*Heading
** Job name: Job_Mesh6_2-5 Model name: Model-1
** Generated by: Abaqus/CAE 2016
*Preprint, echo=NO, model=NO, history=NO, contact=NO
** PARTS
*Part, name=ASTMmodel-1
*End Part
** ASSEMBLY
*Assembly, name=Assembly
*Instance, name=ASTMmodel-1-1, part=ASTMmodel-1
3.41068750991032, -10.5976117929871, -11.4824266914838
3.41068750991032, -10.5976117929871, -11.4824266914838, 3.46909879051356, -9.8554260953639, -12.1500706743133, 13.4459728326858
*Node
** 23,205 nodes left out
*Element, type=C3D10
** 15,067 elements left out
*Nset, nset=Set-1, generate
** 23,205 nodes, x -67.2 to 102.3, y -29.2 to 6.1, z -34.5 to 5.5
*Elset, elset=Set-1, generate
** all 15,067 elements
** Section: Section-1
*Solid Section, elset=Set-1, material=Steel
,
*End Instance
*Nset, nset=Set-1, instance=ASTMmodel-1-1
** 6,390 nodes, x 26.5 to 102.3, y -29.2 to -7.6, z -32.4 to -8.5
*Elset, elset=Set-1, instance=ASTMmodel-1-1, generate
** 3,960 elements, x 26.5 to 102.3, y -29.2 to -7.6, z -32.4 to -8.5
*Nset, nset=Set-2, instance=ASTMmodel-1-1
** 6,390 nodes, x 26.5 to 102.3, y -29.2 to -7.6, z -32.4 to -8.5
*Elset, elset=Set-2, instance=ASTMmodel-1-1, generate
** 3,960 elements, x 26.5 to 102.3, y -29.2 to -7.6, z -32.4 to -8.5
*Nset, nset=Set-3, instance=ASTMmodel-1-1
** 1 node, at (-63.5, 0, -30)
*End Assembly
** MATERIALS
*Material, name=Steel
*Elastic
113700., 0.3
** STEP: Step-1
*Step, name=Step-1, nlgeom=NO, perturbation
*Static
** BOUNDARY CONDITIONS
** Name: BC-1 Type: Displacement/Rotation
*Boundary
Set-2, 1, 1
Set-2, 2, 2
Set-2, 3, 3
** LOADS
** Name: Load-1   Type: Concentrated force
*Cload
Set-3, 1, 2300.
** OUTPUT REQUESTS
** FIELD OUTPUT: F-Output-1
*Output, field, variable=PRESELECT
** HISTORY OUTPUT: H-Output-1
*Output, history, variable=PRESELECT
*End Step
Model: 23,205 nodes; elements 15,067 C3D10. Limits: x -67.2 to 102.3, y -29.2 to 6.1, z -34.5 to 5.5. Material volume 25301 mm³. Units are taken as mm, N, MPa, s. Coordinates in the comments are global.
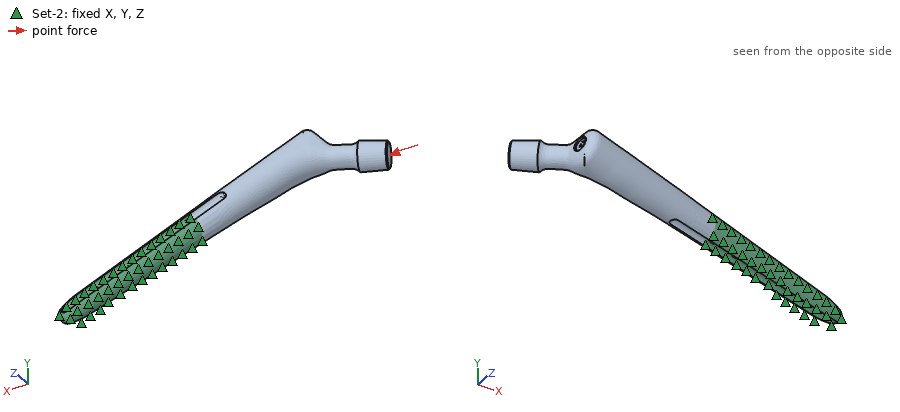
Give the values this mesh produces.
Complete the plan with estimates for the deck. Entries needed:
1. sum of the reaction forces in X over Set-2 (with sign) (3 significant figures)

-2300 N
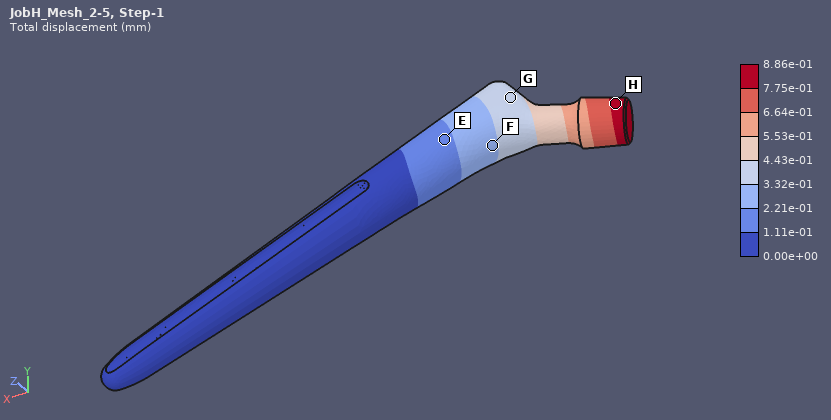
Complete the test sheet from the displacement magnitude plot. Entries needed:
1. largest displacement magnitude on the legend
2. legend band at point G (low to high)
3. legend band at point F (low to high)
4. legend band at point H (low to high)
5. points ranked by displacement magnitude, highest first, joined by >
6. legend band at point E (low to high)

8.86e-01 mm
3.32e-01 to 4.43e-01 mm
2.21e-01 to 3.32e-01 mm
7.75e-01 to 8.86e-01 mm
H > G > F > E
1.11e-01 to 2.21e-01 mm
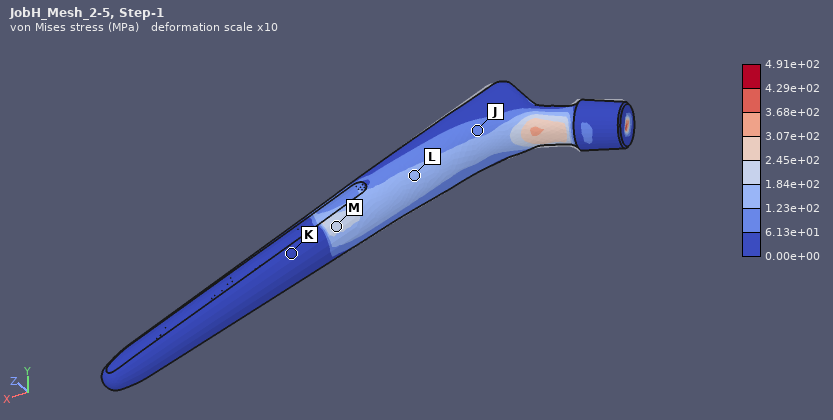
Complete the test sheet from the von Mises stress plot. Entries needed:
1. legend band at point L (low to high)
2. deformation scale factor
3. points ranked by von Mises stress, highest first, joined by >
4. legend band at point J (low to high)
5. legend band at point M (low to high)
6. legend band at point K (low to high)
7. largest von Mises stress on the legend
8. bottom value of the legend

1.23e+02 to 1.84e+02 MPa
10
M > L > J > K
6.13e+01 to 1.23e+02 MPa
1.84e+02 to 2.45e+02 MPa
0.00e+00 to 6.13e+01 MPa
4.91e+02 MPa
0.00e+00 MPa
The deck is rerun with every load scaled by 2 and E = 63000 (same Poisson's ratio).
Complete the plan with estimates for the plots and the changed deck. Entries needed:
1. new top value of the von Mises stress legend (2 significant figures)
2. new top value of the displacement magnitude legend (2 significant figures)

980 MPa
3.2 mm
